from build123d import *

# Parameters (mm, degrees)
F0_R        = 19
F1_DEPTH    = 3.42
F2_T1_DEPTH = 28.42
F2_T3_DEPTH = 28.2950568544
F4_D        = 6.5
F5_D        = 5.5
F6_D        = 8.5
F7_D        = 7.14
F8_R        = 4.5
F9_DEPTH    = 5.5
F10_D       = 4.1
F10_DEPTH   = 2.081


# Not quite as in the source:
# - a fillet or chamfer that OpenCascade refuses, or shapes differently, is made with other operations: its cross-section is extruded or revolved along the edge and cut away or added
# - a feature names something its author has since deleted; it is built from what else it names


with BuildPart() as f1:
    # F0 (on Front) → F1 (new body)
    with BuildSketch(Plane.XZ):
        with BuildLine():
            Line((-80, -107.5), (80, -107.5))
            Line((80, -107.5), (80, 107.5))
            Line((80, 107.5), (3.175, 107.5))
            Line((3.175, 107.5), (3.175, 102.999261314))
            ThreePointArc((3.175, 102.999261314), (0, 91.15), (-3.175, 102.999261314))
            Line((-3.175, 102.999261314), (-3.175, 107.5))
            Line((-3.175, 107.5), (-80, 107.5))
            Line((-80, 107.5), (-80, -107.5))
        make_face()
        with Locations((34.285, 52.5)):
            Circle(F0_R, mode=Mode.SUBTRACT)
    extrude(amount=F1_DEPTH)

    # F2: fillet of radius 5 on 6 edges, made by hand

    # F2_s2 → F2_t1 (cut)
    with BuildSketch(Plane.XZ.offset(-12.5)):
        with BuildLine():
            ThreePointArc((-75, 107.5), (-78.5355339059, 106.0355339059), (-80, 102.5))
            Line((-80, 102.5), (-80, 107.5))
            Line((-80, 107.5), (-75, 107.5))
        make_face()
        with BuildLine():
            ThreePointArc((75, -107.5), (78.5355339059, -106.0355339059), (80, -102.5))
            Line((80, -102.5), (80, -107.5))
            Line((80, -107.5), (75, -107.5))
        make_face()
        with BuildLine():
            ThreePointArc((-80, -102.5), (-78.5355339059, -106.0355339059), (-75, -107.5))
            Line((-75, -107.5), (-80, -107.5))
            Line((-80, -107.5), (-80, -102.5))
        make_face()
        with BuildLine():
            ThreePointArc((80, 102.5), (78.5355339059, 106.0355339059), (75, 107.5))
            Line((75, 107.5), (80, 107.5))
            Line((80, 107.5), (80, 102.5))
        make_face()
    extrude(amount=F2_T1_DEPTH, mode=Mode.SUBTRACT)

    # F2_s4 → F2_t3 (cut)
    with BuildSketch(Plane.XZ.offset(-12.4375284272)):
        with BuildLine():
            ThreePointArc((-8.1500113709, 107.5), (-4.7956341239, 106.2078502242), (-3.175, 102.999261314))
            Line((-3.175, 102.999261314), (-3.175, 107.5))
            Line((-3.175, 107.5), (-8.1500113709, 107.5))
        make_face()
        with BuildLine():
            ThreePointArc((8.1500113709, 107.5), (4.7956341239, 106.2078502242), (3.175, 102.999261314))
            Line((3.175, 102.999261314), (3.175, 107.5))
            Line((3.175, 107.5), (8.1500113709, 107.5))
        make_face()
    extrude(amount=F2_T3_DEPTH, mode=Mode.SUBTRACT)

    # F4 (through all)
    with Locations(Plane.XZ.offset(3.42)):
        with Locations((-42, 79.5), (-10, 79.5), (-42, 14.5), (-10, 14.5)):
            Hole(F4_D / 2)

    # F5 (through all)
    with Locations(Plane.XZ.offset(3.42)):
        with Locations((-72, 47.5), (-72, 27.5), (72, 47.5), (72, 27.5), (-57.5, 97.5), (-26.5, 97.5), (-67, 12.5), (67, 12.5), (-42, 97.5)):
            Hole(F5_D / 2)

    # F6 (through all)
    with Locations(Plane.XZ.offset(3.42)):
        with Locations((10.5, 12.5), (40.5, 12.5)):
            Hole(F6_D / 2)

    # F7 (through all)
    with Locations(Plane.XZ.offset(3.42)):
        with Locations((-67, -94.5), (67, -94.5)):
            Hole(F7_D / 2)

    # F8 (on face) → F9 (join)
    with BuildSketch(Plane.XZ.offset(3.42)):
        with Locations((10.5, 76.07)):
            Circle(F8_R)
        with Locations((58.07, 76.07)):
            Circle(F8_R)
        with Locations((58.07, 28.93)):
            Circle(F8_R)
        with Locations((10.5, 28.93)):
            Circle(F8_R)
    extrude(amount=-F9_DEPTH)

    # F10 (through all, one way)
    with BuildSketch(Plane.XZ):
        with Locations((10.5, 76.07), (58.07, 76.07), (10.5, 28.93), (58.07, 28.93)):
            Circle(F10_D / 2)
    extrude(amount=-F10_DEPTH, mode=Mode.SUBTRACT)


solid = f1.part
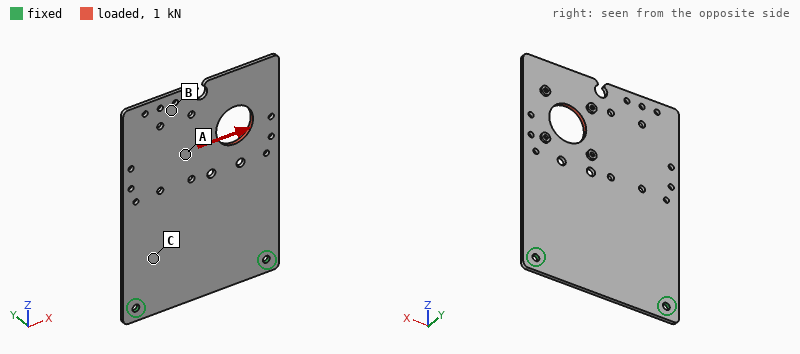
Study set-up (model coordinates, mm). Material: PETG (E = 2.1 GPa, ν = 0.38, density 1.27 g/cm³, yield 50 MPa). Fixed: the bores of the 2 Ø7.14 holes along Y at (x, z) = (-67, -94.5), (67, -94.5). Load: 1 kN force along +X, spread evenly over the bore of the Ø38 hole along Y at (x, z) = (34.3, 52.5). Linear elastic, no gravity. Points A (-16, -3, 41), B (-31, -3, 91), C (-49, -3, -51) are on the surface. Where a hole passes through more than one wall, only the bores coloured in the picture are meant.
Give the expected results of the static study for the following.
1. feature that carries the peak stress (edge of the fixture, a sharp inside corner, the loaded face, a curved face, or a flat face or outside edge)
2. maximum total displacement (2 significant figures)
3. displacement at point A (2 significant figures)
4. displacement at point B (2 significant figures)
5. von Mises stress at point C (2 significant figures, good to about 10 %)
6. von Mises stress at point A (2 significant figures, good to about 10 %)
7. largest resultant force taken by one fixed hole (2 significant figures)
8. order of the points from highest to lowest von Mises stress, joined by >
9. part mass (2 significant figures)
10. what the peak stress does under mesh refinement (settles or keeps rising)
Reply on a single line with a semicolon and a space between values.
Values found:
edge of the fixture; 1.4 mm; 0.87 mm; 1.2 mm; 5.5 MPa; 3.4 MPa; 1.2 kN; C > A > B; 140 g; keeps rising
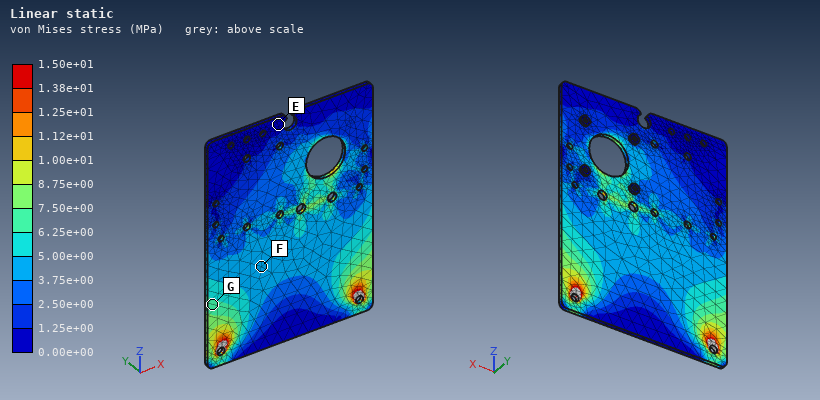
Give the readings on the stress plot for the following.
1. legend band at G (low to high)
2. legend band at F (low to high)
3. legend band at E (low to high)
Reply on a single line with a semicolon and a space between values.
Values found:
6.25e+00 to 7.50e+00 MPa; 3.75e+00 to 5.00e+00 MPa; 0.00e+00 to 1.25e+00 MPa
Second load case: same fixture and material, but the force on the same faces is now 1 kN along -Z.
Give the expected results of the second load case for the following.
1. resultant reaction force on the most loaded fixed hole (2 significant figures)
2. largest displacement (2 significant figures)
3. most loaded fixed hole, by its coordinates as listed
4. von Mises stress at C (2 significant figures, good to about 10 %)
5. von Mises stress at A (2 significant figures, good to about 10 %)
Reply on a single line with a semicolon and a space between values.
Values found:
770 N; 0.46 mm; (67, -94.5); 1.4 MPa; 1.2 MPa
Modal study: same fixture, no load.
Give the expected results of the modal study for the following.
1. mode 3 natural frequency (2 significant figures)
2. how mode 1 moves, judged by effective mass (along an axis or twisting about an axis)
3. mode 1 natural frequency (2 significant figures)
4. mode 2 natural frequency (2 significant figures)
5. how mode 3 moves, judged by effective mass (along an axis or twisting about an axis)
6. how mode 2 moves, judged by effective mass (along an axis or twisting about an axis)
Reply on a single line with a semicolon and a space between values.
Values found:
99 Hz; along Y; 16 Hz; 51 Hz; along Y; twisting about Z
